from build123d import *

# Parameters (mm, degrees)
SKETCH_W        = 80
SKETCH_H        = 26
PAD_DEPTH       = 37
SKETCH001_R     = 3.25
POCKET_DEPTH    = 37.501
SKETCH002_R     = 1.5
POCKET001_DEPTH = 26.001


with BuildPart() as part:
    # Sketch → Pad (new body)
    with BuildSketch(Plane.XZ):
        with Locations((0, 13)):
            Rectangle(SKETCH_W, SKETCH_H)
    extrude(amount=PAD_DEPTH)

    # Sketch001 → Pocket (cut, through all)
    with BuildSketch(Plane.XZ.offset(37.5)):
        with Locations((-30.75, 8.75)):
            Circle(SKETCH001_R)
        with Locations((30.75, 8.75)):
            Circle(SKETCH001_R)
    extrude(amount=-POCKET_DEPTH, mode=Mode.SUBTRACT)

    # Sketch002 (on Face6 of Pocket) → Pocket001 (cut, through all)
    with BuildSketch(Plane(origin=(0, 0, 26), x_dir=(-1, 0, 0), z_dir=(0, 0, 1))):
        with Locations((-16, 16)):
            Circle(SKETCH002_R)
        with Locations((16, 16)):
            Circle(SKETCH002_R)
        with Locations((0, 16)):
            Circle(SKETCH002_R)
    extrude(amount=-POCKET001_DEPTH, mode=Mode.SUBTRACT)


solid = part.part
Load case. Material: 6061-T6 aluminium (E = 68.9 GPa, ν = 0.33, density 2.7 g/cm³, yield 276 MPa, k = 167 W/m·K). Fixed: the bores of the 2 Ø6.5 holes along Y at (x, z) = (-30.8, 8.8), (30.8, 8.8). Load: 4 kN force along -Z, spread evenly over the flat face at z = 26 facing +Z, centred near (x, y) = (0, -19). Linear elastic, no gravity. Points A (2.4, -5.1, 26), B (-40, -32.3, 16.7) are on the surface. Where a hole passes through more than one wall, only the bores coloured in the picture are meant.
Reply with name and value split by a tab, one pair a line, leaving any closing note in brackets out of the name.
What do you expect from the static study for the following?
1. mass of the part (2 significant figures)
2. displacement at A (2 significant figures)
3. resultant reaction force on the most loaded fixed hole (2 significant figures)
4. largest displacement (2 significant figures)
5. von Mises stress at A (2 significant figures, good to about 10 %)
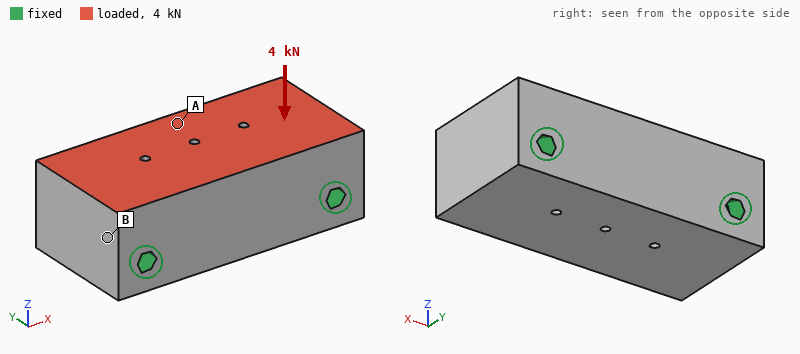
mass of the part	200 g
displacement at A	2.2 µm
resultant reaction force on the most loaded fixed hole	2.1 kN
largest displacement	2.3 µm
von Mises stress at A	3.4 MPa
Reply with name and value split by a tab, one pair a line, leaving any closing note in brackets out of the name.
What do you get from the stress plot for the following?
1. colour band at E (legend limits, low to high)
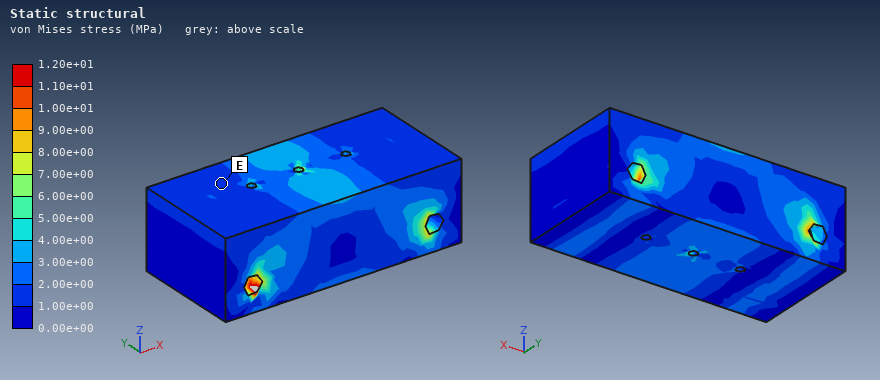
colour band at E	1.00e+00 to 2.00e+00 MPa
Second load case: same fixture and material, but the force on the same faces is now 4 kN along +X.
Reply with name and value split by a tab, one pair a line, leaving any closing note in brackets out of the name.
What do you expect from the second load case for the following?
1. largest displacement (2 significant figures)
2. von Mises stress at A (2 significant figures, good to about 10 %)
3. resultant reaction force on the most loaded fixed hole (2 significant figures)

largest displacement	2.1 µm
von Mises stress at A	2.3 MPa
resultant reaction force on the most loaded fixed hole	2.2 kN
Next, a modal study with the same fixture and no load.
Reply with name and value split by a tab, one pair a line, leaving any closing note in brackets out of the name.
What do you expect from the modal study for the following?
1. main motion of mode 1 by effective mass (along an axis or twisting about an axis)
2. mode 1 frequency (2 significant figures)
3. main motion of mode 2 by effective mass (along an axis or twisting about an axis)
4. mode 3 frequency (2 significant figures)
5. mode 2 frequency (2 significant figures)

main motion of mode 1 by effective mass	along Z
mode 1 frequency	16 kHz
main motion of mode 2 by effective mass	along Y
mode 3 frequency	22 kHz
mode 2 frequency	19 kHz
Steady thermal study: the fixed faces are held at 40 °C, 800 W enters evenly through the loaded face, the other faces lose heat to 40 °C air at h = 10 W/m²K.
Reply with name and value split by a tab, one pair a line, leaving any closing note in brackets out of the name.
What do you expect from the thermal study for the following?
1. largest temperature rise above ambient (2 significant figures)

largest temperature rise above ambient	52 K
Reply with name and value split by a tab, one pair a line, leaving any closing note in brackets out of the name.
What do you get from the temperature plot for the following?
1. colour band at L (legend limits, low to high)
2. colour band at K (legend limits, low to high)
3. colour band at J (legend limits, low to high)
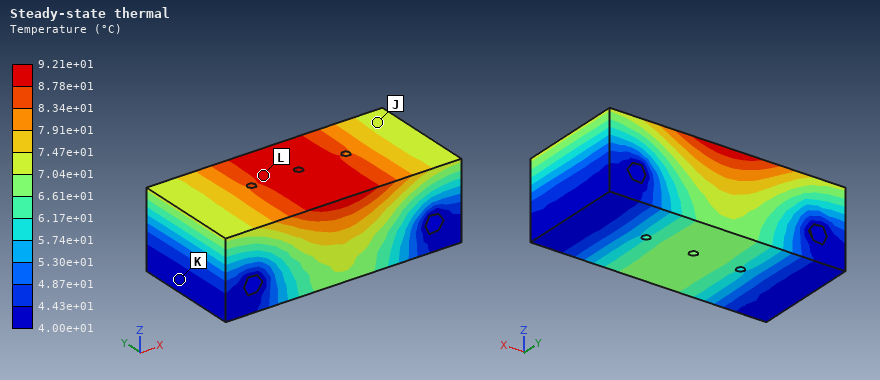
colour band at L	8.78e+01 to 9.21e+01 °C
colour band at K	4.00e+01 to 4.43e+01 °C
colour band at J	7.04e+01 to 7.47e+01 °C
